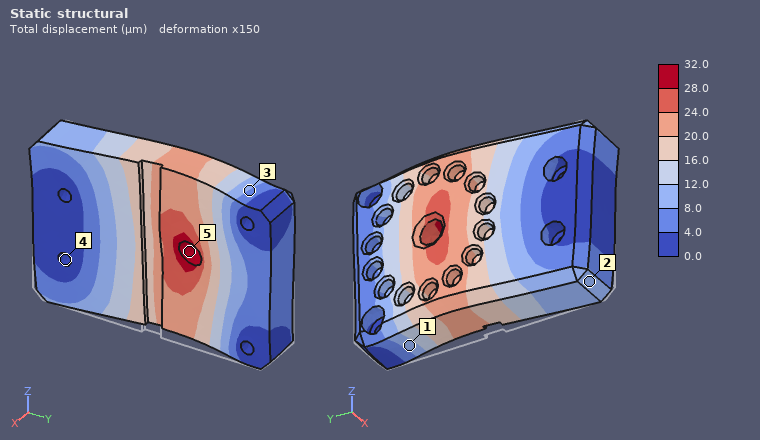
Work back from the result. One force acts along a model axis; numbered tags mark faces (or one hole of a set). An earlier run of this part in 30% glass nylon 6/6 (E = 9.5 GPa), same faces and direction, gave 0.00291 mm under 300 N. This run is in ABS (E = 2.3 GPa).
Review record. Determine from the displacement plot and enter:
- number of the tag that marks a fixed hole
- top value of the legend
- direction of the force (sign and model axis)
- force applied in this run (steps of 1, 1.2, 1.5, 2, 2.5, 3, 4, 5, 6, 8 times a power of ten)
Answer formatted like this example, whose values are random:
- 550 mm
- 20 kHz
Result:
- 4
- 32.0 µm
- +Z
- 800 N
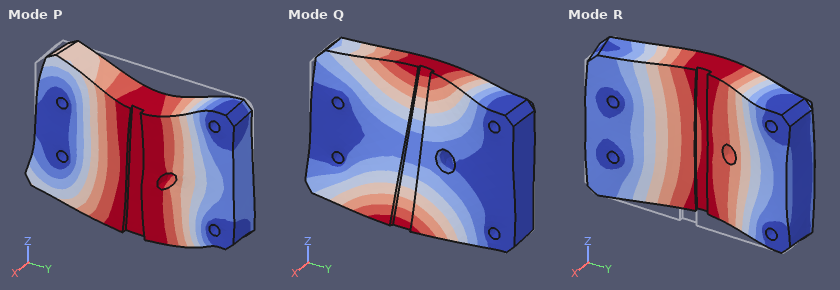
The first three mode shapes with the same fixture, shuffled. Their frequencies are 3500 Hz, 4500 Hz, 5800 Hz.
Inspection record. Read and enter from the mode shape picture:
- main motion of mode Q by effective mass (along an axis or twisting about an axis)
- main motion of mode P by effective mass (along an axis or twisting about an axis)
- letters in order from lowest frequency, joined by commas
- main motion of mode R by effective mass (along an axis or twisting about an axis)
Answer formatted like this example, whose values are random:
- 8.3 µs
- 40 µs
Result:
- twisting about Y
- along Z
- R, Q, P
- along X
